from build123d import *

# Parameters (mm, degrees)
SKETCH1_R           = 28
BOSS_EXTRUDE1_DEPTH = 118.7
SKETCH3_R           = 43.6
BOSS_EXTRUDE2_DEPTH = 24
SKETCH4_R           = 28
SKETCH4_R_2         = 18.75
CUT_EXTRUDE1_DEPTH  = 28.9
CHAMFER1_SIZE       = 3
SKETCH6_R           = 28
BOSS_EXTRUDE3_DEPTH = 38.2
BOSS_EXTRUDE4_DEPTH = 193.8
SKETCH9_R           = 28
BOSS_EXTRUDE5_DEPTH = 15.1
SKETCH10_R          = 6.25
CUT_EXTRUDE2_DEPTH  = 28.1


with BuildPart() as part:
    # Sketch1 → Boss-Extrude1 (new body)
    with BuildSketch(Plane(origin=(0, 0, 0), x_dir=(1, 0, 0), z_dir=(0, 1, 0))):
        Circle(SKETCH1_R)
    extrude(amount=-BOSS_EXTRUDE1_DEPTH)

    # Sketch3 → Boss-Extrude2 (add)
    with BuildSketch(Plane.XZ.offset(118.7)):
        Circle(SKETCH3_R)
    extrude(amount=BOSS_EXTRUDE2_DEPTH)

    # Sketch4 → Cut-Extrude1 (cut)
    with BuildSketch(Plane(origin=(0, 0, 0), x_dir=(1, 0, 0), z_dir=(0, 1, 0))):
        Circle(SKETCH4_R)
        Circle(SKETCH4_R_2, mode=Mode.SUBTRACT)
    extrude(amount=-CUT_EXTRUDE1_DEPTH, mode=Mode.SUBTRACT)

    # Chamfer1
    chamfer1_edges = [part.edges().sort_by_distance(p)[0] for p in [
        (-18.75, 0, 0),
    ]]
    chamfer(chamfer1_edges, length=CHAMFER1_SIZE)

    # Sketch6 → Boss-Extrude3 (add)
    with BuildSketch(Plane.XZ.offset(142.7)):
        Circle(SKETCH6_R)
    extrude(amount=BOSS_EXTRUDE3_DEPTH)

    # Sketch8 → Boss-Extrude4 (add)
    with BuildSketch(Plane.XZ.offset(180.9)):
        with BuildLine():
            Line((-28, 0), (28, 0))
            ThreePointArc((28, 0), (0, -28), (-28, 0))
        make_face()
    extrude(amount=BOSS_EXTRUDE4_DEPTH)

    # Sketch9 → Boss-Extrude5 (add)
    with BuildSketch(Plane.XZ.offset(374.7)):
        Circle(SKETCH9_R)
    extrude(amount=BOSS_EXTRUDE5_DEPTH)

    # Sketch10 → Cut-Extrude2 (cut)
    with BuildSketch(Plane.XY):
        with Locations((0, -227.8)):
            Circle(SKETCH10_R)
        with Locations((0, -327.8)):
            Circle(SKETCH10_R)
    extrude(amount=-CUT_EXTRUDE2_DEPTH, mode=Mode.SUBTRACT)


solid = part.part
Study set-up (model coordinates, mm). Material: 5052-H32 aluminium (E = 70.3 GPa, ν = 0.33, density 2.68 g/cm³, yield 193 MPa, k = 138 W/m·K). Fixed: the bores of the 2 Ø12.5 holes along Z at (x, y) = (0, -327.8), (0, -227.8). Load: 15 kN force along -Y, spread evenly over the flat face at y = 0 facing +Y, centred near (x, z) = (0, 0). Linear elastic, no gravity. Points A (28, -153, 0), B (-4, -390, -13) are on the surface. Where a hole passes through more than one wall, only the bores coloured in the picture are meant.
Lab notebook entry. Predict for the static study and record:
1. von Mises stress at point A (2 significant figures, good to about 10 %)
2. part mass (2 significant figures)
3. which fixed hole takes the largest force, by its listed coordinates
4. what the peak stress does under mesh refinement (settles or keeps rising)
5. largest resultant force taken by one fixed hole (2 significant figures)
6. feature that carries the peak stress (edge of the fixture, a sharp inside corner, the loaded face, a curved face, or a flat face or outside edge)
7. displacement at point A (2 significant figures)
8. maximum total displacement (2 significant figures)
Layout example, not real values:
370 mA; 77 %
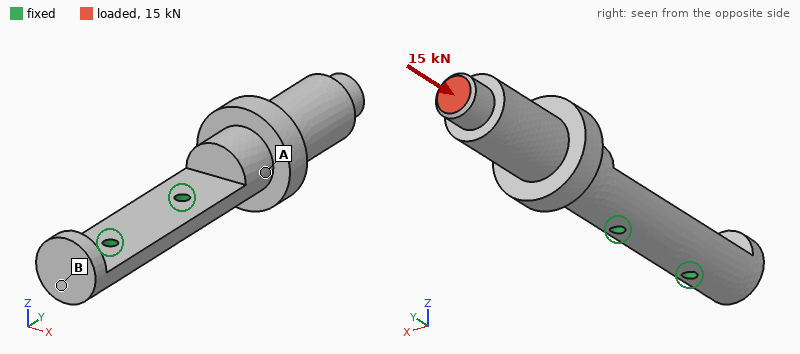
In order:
10 MPa; 2.0 kg; (0, -227.8); keeps rising; 13 kN; edge of the fixture; 0.11 mm; 0.44 mm
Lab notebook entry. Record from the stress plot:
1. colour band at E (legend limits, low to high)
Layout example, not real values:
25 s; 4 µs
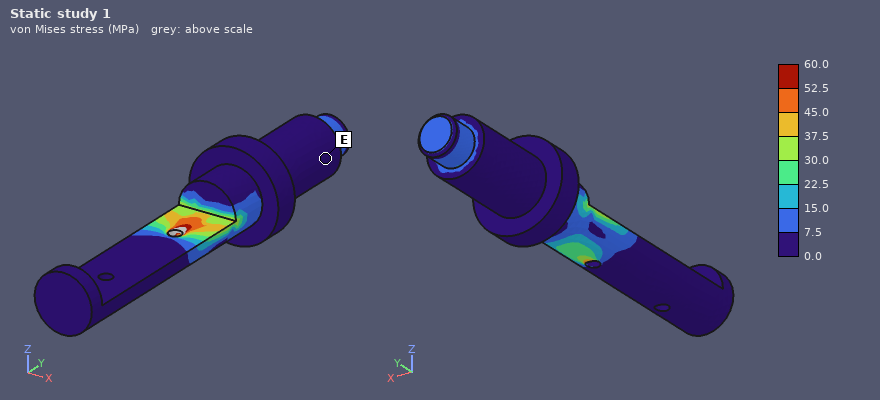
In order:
0.0 to 7.5 MPa
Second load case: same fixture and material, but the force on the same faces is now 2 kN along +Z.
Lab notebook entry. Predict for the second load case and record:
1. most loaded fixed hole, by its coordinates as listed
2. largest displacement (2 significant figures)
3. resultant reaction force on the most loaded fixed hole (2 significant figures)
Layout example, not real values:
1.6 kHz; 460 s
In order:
(0, -227.8); 1.1 mm; 2.8 kN
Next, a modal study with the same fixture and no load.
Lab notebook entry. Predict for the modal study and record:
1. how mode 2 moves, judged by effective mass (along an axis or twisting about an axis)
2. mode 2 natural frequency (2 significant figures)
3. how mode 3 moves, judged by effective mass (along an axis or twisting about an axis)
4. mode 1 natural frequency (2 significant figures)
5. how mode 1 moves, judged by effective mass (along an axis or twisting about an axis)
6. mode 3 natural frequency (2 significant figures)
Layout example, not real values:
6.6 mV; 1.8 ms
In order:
along X; 520 Hz; twisting about Y; 360 Hz; along Z; 1700 Hz
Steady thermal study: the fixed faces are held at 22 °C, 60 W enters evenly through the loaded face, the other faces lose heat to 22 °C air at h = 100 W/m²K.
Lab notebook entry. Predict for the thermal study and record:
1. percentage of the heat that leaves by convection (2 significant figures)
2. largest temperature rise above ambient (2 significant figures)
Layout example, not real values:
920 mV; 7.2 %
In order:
76 %; 31 K
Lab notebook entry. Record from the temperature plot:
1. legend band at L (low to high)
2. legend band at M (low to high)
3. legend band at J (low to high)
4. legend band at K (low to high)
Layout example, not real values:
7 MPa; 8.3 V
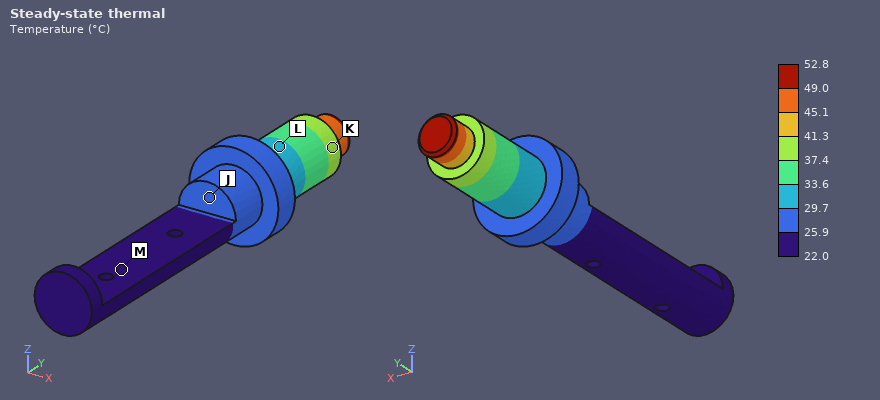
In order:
29.7 to 33.6 °C; 22.0 to 25.9 °C; 25.9 to 29.7 °C; 37.4 to 41.3 °C
